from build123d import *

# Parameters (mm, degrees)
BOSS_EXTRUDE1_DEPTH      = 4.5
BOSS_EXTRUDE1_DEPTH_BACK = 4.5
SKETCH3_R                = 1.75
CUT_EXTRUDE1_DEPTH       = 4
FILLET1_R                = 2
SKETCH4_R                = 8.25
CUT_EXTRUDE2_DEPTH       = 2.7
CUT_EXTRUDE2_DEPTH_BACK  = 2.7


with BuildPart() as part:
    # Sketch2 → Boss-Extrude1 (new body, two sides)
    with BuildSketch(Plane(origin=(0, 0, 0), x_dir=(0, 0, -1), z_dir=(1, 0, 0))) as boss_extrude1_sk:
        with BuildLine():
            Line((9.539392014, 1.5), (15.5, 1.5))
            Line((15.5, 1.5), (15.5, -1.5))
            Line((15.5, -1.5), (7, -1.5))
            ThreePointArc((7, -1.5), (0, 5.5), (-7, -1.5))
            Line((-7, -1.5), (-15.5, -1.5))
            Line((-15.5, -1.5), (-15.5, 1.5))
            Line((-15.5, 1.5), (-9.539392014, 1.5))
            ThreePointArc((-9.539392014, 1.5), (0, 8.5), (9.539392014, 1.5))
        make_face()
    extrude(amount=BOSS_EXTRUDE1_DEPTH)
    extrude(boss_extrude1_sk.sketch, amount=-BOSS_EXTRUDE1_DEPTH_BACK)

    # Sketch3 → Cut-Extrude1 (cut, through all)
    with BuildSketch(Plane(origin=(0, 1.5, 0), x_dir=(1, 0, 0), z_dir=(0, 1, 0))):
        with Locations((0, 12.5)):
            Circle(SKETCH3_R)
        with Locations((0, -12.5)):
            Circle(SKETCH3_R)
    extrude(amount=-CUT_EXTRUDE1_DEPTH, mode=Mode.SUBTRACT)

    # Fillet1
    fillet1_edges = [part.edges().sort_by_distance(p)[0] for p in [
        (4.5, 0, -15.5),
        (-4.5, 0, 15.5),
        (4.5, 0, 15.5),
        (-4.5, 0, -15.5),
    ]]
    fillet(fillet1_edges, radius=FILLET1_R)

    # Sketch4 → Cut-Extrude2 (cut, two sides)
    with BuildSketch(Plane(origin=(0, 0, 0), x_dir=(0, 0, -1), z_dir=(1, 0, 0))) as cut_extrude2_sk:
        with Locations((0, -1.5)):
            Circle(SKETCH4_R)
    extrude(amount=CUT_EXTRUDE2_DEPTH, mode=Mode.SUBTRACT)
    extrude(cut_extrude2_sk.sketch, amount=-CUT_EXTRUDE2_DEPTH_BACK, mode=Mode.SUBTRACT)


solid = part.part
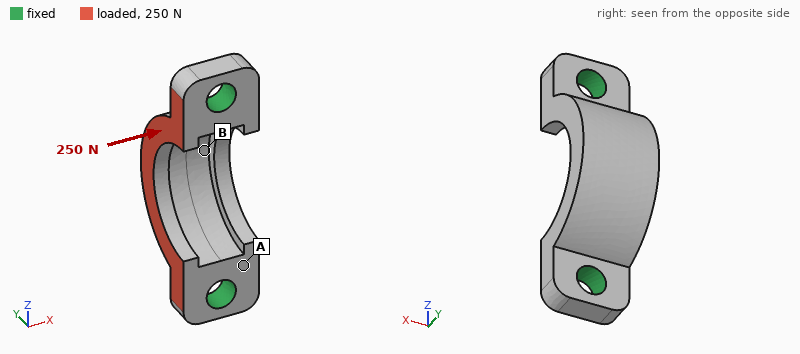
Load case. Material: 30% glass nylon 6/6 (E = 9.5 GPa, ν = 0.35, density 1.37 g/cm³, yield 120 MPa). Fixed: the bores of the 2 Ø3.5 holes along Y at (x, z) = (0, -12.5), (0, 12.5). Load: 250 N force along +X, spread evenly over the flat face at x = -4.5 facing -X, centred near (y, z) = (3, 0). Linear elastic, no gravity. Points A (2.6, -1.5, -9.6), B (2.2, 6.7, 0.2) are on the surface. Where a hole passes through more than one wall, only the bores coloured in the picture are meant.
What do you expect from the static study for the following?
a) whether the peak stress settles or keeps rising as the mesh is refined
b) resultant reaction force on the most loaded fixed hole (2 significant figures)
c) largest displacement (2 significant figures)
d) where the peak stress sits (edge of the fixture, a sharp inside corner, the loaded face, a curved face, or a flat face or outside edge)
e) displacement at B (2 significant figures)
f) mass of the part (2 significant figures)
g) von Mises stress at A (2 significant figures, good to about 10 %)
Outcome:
keeps rising
130 N
63 µm
edge of the fixture
48 µm
1.1 g
8.6 MPa
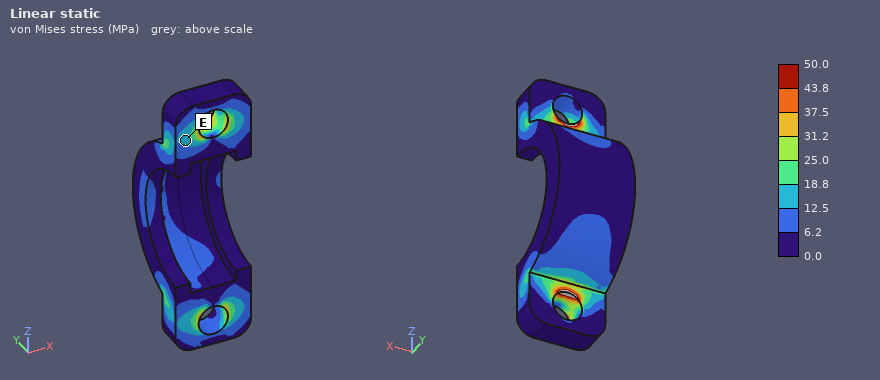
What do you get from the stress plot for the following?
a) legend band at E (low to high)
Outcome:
12.5 to 18.8 MPa
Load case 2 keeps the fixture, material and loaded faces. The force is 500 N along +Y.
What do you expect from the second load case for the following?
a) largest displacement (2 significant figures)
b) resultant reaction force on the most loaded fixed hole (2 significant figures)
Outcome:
0.15 mm
270 N
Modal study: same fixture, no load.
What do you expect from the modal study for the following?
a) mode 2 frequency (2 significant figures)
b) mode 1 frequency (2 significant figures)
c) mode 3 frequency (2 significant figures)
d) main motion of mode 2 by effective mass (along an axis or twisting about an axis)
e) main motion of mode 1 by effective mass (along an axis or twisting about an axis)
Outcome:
18 kHz
12 kHz
24 kHz
along Z
along X
